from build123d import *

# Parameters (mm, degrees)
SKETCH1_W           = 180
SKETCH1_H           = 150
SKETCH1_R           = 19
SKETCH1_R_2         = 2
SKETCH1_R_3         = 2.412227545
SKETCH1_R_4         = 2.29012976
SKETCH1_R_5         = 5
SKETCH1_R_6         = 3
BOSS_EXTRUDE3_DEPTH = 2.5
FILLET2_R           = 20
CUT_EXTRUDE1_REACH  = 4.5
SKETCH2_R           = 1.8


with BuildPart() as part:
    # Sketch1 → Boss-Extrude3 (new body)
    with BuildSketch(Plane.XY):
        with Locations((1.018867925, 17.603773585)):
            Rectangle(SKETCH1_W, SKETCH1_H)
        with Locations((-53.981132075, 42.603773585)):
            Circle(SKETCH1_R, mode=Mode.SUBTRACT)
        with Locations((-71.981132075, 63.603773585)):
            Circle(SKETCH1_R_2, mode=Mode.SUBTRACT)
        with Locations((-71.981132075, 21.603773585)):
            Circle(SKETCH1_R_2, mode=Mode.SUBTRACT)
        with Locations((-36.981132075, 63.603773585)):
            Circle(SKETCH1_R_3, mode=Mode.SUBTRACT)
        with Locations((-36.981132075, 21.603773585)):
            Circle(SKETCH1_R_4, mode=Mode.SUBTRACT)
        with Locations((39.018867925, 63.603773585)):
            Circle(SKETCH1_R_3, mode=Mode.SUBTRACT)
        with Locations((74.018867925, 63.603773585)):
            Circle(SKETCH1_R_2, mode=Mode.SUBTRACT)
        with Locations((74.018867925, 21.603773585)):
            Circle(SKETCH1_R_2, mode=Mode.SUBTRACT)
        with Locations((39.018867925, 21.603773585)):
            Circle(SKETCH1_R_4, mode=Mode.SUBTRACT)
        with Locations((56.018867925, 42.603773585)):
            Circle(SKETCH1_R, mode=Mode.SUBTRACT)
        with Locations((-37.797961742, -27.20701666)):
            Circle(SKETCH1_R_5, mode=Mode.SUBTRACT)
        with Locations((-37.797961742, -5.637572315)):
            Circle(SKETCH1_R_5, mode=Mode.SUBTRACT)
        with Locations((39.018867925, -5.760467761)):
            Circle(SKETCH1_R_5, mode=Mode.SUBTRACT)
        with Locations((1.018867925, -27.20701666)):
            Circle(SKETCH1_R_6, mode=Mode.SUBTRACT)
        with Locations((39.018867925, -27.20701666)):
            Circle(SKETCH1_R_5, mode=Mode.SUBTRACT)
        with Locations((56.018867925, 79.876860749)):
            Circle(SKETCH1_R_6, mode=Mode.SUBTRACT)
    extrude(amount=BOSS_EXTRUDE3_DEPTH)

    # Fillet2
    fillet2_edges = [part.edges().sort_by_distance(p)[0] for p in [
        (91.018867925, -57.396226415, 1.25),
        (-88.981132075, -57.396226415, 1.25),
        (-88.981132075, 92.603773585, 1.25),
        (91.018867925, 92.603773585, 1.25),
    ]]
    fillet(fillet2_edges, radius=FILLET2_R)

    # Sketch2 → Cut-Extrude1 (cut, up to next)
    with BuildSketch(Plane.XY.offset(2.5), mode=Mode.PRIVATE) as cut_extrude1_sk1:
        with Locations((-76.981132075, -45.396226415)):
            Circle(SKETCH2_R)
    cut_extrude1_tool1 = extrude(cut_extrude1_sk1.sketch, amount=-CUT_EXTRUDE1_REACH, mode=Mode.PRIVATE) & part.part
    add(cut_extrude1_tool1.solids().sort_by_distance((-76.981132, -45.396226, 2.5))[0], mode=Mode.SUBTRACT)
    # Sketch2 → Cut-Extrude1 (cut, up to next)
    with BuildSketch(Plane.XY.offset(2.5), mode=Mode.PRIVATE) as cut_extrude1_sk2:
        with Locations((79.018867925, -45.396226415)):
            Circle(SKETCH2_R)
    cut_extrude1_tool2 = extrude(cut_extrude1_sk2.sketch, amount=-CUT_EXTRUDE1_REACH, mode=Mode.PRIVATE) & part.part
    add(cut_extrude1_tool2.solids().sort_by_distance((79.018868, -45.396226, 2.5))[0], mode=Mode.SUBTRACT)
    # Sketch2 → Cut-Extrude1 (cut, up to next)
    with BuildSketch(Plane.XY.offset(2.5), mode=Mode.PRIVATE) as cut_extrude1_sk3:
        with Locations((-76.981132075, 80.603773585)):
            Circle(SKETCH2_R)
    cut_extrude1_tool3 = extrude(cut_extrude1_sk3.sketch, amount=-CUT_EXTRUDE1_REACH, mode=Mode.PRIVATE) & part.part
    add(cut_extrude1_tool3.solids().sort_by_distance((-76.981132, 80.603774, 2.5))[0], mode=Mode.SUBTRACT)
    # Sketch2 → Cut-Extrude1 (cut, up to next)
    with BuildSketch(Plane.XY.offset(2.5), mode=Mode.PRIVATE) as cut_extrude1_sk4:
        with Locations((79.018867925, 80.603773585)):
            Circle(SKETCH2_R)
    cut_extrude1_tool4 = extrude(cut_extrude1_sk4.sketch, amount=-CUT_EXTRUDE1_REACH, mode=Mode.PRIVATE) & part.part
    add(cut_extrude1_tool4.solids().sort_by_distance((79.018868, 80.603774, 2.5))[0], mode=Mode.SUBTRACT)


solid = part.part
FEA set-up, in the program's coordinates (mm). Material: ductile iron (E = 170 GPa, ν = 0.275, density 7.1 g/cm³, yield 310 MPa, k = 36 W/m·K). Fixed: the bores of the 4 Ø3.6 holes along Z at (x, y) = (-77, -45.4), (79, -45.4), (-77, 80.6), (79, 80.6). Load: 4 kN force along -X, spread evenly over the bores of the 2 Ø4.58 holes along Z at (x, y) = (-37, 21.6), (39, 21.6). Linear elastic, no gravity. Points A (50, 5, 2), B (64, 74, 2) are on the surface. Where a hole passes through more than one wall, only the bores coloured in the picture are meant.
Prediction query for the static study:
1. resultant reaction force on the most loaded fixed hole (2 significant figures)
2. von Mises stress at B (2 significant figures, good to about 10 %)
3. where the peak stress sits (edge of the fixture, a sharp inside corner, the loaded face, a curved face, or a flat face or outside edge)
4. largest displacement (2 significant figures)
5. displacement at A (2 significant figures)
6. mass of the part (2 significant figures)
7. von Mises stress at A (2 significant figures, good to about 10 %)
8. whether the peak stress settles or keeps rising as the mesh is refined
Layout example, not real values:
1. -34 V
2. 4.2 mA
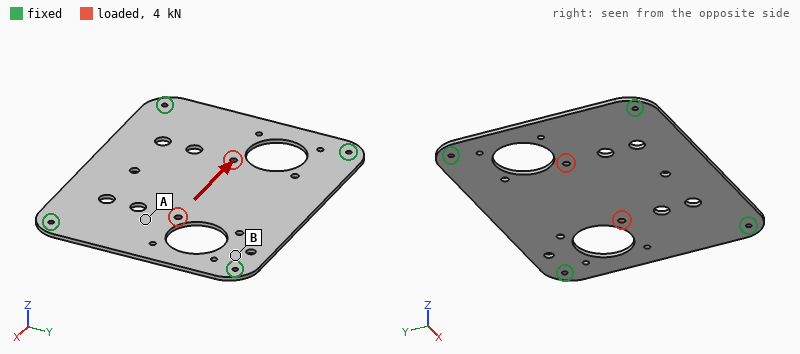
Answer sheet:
1. 1.3 kN
2. 19 MPa
3. edge of the fixture
4. 13 µm
5. 8.9 µm
6. 420 g
7. 6.1 MPa
8. keeps rising
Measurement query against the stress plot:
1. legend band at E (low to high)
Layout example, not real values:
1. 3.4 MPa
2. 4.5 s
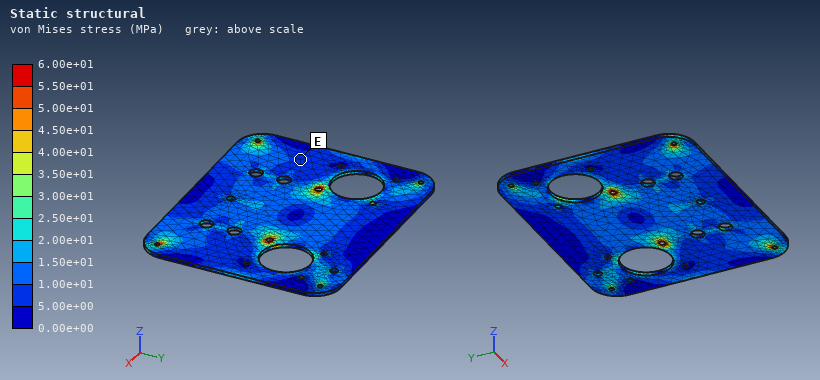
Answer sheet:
1. 5.00e+00 to 1.00e+01 MPa
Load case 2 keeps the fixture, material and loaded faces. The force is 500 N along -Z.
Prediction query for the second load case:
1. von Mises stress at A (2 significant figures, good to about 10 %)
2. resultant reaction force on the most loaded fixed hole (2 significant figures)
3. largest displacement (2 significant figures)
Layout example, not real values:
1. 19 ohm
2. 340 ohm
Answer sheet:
1. 32 MPa
2. 140 N
3. 0.54 mm
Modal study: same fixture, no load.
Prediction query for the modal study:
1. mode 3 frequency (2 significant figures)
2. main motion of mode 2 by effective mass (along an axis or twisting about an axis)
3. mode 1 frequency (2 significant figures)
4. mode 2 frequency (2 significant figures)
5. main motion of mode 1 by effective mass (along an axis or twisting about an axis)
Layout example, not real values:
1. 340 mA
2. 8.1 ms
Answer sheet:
1. 760 Hz
2. twisting about X
3. 370 Hz
4. 580 Hz
5. along Z
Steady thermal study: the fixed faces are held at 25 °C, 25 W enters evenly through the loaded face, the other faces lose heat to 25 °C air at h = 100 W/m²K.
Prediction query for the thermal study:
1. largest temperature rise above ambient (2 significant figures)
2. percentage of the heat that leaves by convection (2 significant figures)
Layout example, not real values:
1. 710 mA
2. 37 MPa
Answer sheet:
1. 64 K
2. 98 %
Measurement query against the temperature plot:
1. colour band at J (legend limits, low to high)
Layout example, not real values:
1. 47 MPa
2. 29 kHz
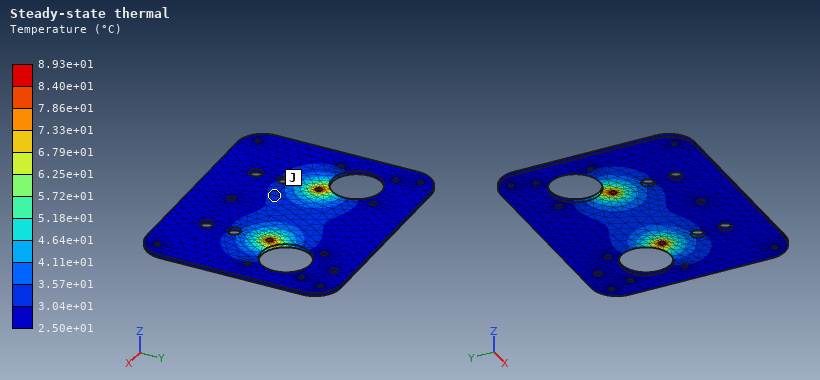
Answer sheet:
1. 3.04e+01 to 3.57e+01 °C
